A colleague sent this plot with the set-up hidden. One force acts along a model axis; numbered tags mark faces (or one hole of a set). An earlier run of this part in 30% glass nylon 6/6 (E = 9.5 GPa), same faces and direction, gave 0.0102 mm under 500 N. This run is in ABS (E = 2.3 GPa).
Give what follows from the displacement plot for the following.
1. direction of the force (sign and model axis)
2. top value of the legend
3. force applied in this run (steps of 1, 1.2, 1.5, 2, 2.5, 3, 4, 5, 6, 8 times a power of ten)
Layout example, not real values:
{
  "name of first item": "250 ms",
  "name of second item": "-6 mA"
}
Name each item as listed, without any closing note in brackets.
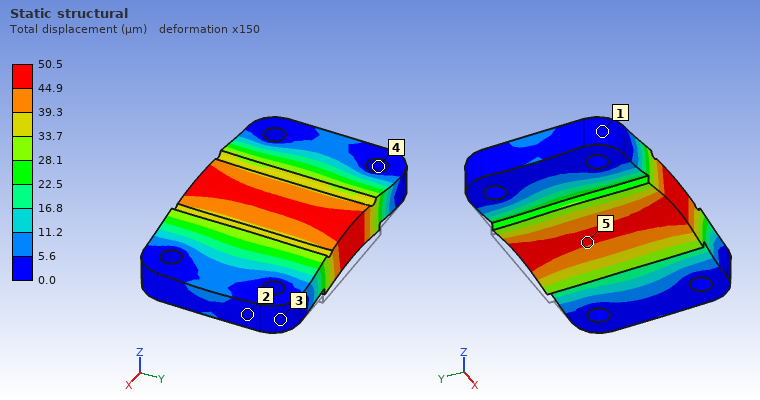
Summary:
{
  "direction of the force": "+Z",
  "top value of the legend": "50.5 µm",
  "force applied in this run": "600 N"
}
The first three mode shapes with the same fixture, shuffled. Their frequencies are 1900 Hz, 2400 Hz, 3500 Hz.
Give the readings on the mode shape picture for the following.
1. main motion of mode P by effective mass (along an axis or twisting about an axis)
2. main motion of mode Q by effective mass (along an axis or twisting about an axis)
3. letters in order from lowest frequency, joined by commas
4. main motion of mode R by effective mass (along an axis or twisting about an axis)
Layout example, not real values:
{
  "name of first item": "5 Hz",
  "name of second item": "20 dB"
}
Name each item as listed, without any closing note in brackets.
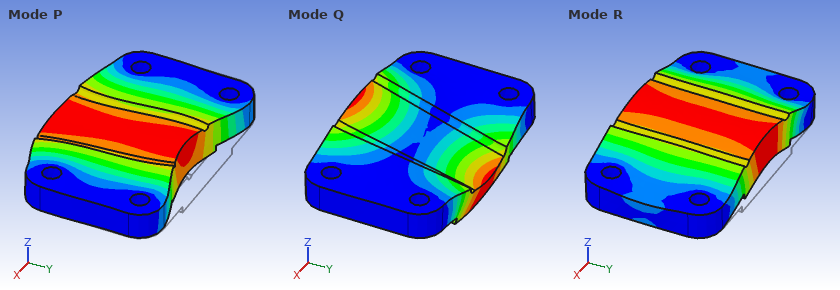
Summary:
{
  "main motion of mode P by effective mass": "along Y",
  "main motion of mode Q by effective mass": "twisting about X",
  "letters in order from lowest frequency, joined by commas": "R, Q, P",
  "main motion of mode R by effective mass": "along Z"
}
